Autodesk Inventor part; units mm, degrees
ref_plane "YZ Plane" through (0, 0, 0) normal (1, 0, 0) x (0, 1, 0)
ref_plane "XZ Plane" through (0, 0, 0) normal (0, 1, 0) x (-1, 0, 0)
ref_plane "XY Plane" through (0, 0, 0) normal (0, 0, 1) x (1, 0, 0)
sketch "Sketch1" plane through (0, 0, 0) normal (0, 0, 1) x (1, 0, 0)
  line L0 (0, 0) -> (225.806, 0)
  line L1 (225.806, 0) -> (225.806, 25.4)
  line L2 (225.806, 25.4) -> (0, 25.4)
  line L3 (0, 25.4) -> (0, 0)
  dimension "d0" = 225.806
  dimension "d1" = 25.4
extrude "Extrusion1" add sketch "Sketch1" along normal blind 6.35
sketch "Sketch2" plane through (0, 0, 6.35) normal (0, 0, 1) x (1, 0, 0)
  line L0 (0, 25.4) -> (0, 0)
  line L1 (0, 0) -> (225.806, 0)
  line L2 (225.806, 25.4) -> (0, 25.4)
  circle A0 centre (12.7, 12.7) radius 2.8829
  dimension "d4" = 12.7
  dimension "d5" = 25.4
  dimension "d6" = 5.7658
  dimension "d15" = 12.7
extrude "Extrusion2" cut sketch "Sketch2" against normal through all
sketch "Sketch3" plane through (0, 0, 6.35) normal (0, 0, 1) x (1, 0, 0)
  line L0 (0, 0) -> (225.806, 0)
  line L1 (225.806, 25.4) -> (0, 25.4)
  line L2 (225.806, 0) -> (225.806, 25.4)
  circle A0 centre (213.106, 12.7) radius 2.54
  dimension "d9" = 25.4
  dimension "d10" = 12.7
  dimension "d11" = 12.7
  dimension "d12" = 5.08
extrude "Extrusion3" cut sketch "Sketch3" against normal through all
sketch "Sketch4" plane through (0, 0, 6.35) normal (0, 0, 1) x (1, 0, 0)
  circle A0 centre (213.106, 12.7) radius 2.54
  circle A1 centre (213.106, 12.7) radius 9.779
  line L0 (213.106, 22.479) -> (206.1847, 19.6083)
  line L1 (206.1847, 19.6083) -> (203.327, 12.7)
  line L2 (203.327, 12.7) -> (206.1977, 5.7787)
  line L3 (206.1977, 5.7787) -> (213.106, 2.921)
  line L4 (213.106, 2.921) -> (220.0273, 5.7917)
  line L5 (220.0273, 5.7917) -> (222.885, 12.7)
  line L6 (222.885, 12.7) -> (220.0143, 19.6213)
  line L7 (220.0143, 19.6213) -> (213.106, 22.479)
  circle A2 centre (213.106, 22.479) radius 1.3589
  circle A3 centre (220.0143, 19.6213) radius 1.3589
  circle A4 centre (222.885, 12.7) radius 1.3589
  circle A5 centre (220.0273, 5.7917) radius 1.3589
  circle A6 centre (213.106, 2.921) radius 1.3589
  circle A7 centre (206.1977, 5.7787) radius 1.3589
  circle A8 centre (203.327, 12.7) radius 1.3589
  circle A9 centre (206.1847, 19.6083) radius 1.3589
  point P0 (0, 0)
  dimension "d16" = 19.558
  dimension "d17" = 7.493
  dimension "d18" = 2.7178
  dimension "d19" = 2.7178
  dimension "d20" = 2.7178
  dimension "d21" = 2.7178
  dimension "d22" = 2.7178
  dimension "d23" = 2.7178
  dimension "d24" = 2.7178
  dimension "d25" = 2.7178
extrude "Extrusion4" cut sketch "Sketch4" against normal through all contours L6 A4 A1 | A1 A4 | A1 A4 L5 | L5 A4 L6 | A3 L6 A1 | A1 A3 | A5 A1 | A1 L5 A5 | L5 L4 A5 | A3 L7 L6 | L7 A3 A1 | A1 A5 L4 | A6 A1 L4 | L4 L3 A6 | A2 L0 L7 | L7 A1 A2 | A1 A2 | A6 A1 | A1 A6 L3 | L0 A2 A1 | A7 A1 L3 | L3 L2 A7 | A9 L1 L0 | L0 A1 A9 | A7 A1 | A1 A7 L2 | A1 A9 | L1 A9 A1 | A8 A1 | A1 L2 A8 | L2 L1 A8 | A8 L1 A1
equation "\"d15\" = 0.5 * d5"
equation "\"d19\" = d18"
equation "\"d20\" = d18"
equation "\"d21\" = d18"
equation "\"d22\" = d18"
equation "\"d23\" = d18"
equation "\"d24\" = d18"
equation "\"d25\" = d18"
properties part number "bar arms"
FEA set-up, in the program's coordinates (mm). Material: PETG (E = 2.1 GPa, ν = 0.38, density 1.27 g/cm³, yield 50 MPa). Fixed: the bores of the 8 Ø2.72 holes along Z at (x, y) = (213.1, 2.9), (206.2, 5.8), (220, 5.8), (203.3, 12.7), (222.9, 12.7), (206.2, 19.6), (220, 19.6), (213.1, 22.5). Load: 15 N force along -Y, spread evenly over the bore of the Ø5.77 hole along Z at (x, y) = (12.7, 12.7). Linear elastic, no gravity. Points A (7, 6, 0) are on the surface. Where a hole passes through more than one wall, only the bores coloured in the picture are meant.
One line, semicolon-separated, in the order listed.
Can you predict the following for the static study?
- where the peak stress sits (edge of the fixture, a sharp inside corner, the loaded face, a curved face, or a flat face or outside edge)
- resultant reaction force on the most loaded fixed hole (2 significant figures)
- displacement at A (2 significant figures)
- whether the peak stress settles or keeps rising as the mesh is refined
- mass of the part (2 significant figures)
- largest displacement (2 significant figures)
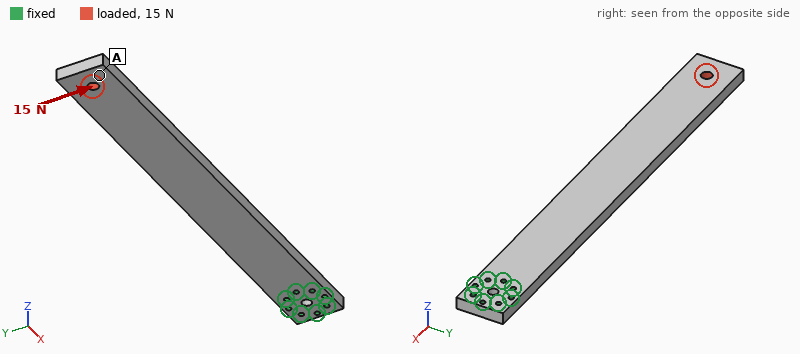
edge of the fixture; 120 N; 2.2 mm; keeps rising; 46 g; 2.3 mm
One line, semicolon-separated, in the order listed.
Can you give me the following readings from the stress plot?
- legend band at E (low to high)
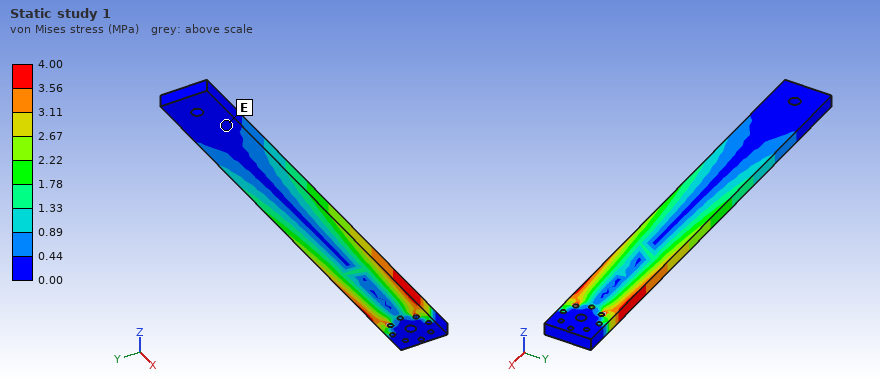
0.00 to 0.44 MPa
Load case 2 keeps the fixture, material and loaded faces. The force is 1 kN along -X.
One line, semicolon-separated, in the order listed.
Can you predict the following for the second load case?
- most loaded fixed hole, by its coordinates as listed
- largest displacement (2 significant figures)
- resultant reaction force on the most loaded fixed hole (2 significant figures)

(203.3, 12.7); 0.61 mm; 330 N
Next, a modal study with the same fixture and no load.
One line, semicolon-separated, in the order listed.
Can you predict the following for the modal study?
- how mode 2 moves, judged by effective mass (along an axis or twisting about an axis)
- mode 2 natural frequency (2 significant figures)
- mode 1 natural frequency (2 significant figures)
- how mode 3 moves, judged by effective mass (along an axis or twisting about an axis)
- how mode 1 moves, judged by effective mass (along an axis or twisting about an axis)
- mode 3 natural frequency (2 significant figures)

along Y; 120 Hz; 32 Hz; along Z; along Z; 200 Hz
